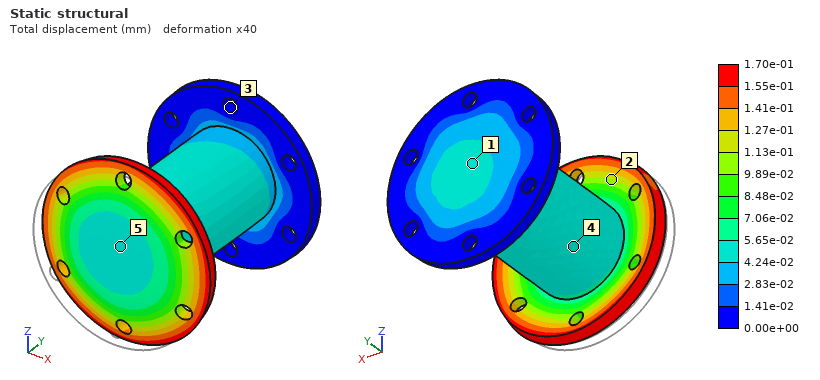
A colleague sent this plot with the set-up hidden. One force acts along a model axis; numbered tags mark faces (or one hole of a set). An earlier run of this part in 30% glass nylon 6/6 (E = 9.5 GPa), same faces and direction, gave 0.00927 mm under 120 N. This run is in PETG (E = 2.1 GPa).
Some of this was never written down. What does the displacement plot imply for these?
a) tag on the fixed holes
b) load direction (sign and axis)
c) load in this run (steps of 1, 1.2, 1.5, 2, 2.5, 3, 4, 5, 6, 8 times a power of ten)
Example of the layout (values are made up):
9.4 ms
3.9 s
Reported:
3
+Y
500 N
